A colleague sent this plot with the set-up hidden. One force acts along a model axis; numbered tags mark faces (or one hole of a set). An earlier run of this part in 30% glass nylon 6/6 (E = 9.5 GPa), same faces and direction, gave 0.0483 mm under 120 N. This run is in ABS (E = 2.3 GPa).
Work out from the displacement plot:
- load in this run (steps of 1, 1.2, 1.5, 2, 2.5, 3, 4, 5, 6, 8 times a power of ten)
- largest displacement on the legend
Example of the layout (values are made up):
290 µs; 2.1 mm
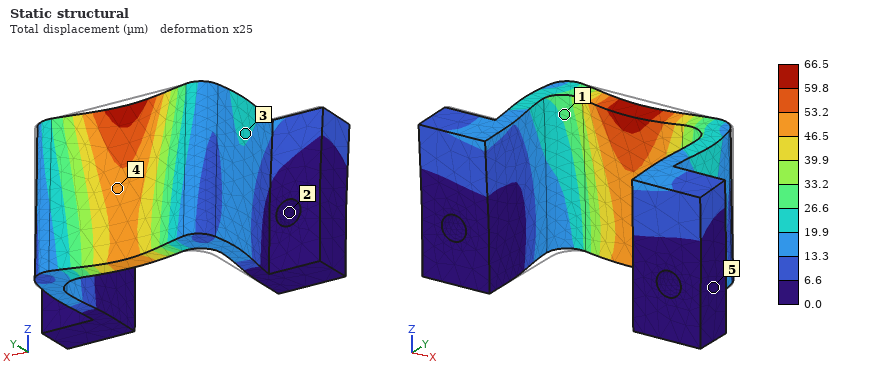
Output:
40 N; 66.5 µm
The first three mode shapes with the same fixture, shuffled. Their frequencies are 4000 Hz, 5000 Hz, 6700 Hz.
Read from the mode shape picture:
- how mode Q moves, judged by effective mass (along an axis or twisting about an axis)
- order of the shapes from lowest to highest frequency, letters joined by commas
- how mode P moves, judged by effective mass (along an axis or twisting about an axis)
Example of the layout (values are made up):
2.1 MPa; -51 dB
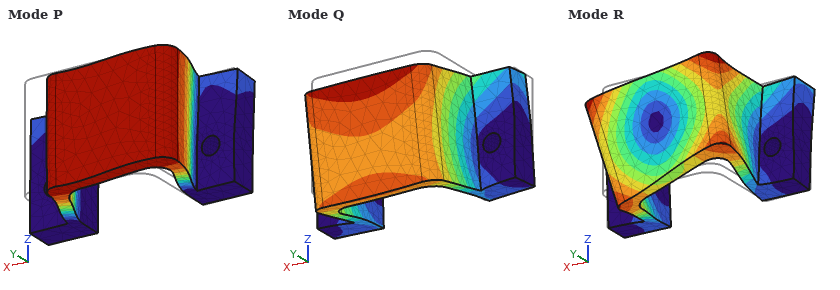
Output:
along Z; P, Q, R; along X
